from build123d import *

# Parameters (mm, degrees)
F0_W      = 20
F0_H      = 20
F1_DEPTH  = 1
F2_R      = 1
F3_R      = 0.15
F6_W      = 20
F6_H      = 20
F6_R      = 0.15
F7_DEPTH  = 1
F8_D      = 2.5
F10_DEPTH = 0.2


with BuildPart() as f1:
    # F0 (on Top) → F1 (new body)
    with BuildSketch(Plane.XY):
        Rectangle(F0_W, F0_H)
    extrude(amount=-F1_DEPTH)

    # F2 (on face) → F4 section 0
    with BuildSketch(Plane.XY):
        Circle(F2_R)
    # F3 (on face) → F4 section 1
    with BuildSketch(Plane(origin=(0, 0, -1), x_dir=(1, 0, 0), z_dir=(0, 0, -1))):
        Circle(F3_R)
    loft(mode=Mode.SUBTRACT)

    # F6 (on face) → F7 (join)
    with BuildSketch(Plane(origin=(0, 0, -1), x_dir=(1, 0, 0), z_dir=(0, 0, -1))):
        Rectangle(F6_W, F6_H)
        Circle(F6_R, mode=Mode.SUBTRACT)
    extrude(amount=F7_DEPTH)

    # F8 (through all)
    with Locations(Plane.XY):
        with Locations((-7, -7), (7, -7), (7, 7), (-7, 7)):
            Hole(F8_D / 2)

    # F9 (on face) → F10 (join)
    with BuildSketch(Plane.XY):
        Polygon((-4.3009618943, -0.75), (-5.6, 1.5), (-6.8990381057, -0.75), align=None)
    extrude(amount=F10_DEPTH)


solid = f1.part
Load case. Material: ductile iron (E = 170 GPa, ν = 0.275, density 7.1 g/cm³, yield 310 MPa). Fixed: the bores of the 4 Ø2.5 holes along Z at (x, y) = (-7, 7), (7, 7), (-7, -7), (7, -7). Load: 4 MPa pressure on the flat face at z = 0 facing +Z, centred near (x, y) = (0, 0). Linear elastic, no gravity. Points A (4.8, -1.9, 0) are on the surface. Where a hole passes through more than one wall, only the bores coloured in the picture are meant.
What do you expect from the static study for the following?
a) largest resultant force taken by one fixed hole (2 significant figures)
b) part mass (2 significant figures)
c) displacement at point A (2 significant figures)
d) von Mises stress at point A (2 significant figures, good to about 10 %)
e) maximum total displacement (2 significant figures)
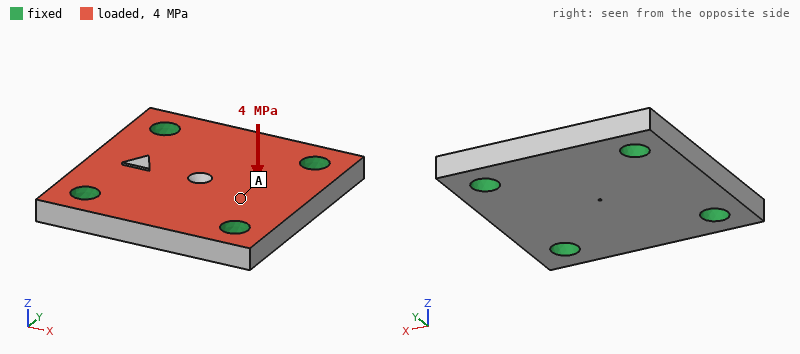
380 N
5.4 g
4.4 µm
33 MPa
6.8 µm
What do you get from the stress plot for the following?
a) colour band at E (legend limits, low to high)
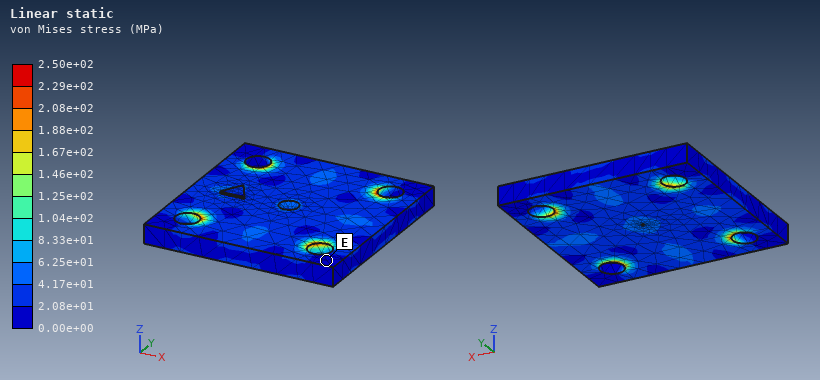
0.00e+00 to 2.08e+01 MPa
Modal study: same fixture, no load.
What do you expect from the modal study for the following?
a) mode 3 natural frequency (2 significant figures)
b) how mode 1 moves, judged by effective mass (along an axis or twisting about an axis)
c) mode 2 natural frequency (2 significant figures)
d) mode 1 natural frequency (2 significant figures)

58 kHz
along Z
58 kHz
39 kHz
